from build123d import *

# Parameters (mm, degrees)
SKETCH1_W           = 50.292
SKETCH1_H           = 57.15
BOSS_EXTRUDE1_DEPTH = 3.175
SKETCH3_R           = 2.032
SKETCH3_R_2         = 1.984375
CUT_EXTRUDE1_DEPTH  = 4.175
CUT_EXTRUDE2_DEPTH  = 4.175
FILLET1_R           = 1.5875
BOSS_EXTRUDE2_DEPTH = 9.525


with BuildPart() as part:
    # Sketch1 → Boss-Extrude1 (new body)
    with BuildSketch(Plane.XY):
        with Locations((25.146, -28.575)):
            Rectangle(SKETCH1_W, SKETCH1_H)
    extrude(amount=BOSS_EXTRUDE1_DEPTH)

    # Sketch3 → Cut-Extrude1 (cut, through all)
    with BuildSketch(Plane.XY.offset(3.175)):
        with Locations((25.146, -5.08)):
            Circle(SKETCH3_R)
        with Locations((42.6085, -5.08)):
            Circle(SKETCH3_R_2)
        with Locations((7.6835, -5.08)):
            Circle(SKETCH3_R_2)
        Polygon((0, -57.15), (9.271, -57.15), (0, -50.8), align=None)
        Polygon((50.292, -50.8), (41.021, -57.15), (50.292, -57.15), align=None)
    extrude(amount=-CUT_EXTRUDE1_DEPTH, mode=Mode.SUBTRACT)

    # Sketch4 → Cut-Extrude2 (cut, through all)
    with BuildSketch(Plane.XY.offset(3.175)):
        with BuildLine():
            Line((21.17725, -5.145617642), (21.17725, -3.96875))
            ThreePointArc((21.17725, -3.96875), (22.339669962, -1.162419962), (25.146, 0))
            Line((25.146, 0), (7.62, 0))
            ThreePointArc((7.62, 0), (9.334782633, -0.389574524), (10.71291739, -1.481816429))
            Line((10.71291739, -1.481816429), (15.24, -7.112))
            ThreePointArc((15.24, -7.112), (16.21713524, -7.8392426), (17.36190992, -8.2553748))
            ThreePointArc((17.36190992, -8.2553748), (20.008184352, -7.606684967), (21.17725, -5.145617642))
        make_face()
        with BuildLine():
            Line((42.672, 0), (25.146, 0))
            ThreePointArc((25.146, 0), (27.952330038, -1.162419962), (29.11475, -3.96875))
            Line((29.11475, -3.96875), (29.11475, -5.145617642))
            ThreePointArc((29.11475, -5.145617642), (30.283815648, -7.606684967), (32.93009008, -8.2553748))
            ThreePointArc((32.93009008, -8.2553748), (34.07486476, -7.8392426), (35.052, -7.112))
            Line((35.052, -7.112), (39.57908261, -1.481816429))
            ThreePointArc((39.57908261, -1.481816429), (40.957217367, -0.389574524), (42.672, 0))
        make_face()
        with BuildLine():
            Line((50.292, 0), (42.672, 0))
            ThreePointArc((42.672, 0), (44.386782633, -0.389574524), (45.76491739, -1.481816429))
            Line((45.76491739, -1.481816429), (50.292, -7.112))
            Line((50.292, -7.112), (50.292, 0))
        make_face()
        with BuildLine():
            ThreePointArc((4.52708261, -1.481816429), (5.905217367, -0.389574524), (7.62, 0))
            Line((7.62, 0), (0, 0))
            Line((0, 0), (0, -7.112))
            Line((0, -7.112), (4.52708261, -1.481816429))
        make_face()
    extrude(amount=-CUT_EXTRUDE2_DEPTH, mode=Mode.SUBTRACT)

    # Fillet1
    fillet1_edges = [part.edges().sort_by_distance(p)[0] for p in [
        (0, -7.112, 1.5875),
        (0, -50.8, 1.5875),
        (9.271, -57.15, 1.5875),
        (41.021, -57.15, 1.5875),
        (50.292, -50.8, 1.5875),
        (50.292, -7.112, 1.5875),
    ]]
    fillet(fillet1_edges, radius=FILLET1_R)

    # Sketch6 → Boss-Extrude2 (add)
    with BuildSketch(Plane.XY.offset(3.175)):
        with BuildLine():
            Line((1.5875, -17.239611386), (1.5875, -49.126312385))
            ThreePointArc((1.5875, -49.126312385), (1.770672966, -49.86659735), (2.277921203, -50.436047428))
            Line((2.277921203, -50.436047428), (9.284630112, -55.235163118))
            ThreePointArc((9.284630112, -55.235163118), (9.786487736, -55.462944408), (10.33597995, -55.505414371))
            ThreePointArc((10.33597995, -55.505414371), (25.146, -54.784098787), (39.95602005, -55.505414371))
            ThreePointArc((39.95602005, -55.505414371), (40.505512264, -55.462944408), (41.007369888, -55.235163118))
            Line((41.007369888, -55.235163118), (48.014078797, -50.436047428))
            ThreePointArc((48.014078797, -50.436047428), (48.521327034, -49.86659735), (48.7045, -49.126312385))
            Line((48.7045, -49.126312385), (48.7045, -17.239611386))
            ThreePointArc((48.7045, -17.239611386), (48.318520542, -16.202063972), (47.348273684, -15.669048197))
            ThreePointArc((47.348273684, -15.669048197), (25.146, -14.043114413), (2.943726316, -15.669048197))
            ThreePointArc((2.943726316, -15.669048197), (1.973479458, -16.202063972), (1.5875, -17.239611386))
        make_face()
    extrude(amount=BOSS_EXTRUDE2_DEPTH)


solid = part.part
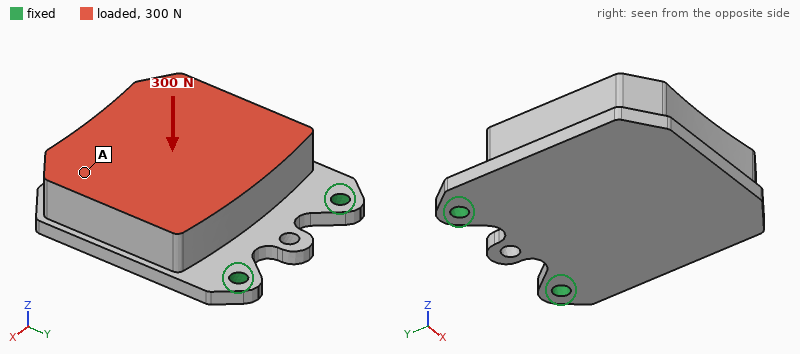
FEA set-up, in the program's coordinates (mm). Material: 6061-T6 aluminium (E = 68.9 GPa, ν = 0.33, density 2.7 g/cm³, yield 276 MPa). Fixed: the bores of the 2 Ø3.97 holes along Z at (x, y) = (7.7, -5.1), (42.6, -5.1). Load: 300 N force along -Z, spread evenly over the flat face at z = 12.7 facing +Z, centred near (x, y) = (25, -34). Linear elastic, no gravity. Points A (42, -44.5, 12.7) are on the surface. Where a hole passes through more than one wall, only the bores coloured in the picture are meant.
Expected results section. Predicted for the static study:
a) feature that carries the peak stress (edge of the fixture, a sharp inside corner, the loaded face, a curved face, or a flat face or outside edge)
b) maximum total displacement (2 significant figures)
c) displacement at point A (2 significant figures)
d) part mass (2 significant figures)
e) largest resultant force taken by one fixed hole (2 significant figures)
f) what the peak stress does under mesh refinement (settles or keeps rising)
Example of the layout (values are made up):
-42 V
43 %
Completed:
edge of the fixture
0.57 mm
0.44 mm
70 g
150 N
keeps rising
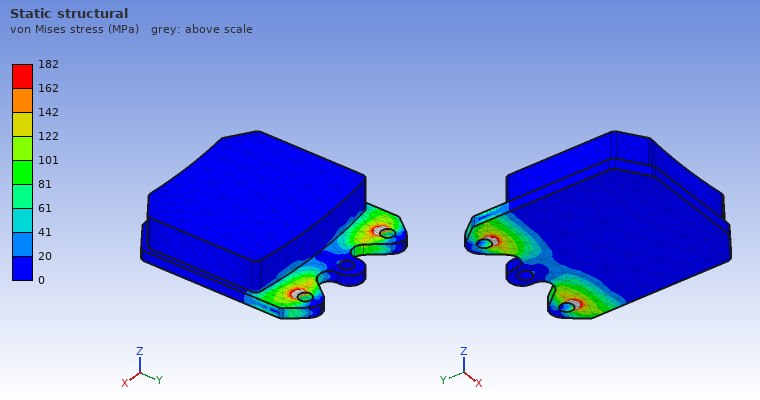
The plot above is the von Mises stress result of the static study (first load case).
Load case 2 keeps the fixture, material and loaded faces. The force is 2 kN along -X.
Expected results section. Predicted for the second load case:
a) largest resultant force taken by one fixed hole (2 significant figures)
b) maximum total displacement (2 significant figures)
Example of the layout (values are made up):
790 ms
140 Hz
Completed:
1.9 kN
65 µm
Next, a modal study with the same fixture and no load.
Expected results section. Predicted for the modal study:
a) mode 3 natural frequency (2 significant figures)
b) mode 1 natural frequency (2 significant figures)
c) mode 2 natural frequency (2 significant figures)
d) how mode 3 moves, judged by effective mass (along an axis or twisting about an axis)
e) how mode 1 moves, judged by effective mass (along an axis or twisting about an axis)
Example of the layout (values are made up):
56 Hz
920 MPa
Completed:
5400 Hz
550 Hz
4100 Hz
along X
along Z
